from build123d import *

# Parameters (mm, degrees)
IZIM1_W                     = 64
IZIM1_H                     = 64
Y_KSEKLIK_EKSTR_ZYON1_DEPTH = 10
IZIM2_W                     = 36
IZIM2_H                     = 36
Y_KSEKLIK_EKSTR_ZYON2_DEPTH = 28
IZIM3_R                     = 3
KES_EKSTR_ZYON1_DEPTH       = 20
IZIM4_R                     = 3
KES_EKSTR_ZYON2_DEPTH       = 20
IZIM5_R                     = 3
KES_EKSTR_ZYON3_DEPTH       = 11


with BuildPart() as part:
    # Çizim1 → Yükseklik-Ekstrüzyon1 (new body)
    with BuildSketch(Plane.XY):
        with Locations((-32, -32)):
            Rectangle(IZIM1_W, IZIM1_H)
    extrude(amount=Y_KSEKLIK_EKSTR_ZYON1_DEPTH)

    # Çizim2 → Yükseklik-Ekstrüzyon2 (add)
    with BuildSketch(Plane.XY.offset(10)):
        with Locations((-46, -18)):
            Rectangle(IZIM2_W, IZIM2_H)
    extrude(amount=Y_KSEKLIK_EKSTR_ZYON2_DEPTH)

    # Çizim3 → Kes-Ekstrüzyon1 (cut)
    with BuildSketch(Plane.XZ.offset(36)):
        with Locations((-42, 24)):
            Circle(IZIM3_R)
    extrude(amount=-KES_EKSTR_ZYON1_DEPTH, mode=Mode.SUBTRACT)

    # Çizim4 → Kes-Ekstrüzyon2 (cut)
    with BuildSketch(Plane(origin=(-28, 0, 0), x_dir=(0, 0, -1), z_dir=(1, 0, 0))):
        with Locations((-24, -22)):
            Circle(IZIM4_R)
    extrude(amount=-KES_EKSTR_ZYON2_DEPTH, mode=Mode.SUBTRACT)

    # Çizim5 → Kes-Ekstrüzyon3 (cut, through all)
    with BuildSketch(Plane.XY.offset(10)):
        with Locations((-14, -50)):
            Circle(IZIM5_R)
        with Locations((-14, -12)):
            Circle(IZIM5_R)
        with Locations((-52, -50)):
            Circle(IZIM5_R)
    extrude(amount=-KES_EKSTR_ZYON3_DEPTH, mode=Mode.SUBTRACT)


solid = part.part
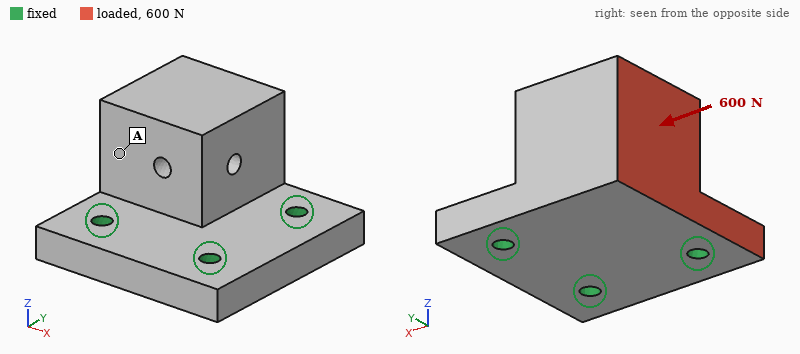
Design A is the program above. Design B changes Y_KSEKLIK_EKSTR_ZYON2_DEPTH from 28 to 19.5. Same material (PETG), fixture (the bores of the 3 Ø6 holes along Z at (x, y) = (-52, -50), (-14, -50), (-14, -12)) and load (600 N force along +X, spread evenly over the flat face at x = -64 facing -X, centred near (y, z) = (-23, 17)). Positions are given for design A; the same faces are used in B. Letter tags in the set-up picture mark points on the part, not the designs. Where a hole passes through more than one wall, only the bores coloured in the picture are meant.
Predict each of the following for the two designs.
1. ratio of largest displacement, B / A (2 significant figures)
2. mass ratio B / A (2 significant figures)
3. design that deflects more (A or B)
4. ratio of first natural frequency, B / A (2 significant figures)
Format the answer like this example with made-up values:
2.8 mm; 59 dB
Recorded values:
0.63; 0.85; A; 1.3
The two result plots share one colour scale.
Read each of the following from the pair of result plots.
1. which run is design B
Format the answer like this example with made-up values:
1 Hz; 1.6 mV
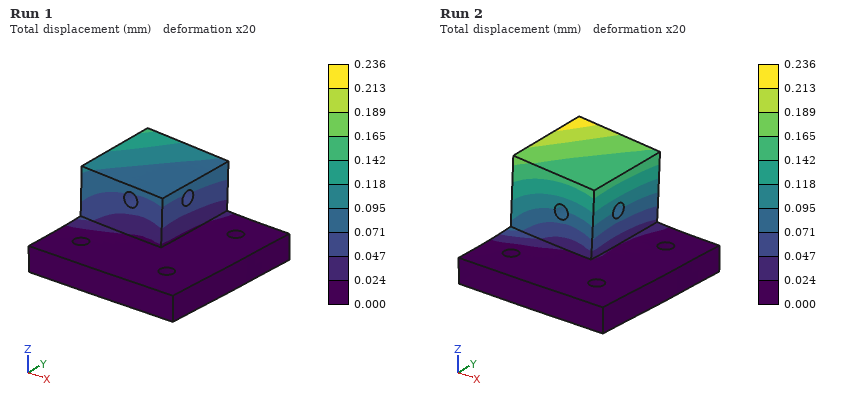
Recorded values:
Run 1
